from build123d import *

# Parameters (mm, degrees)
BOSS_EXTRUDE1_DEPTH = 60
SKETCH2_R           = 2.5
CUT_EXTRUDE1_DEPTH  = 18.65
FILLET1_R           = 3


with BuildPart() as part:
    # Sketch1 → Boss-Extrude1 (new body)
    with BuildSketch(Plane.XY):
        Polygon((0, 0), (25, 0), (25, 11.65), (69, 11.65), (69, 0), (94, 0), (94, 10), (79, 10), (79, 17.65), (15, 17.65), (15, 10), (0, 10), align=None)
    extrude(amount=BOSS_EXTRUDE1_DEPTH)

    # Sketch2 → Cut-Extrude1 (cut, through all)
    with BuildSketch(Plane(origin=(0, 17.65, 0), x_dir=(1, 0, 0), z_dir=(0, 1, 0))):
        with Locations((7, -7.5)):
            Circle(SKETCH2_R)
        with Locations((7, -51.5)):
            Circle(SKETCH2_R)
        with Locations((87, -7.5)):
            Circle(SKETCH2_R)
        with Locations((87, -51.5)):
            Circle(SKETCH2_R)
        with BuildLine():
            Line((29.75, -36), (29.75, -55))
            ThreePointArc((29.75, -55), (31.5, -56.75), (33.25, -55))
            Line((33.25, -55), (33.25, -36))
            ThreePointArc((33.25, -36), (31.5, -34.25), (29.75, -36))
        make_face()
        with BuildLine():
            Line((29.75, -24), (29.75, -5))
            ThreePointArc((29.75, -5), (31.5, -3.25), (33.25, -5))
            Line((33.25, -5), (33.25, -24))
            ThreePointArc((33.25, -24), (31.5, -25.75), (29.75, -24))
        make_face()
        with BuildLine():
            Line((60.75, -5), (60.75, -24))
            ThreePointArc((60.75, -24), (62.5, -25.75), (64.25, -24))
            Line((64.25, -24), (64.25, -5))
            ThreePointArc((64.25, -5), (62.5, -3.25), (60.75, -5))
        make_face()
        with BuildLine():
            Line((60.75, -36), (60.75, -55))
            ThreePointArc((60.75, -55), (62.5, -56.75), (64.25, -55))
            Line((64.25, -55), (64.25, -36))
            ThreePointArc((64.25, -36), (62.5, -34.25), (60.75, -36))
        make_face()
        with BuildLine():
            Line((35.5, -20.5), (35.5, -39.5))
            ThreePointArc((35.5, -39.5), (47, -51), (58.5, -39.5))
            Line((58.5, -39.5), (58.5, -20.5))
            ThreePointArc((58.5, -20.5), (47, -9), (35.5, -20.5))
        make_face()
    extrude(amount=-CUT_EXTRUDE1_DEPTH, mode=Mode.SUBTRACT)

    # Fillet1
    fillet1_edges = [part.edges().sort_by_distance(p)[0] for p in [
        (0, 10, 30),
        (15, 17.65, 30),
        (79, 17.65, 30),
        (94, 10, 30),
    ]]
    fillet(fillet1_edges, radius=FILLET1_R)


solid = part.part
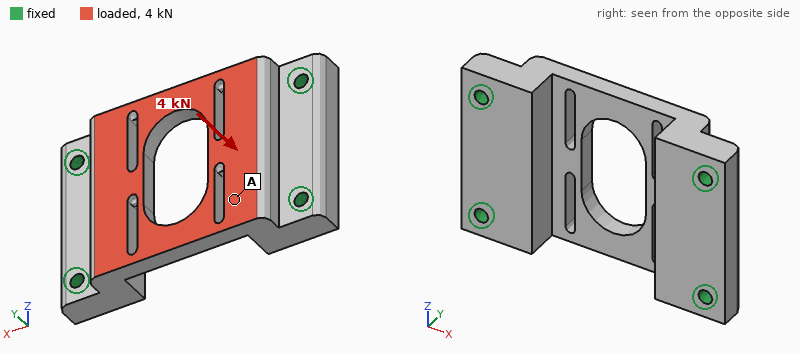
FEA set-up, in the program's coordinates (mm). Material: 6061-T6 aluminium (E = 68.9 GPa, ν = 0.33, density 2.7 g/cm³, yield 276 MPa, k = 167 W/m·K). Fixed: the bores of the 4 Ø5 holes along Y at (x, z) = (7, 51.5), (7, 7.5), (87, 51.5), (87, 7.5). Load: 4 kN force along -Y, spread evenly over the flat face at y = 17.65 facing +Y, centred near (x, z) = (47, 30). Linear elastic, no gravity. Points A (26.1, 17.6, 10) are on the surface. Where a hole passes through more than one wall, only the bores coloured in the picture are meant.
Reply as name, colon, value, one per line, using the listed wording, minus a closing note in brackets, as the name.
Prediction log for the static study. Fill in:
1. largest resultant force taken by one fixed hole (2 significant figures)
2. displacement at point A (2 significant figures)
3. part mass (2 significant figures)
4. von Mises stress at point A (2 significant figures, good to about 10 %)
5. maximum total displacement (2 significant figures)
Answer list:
largest resultant force taken by one fixed hole: 1.2 kN
displacement at point A: 22 µm
part mass: 130 g
von Mises stress at point A: 10 MPa
maximum total displacement: 56 µm
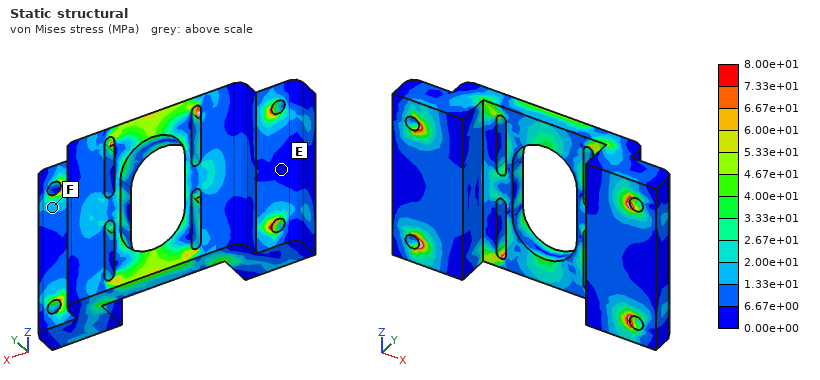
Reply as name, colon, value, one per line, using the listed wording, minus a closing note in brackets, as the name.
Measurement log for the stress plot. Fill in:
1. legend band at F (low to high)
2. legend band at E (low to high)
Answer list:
legend band at F: 1.33e+01 to 2.00e+01 MPa
legend band at E: 0.00e+00 to 6.67e+00 MPa
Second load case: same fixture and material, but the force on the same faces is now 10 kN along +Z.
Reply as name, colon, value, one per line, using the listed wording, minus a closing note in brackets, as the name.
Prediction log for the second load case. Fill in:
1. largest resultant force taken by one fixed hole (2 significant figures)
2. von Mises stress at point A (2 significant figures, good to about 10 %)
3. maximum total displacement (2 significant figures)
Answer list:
largest resultant force taken by one fixed hole: 3.5 kN
von Mises stress at point A: 26 MPa
maximum total displacement: 49 µm
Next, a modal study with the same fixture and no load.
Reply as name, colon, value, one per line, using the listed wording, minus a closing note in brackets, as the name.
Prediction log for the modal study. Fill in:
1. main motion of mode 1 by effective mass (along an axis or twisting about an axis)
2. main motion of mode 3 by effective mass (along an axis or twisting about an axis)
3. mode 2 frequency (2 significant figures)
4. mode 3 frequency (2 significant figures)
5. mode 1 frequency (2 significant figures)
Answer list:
main motion of mode 1 by effective mass: along Y
main motion of mode 3 by effective mass: twisting about X
mode 2 frequency: 8600 Hz
mode 3 frequency: 9400 Hz
mode 1 frequency: 7700 Hz
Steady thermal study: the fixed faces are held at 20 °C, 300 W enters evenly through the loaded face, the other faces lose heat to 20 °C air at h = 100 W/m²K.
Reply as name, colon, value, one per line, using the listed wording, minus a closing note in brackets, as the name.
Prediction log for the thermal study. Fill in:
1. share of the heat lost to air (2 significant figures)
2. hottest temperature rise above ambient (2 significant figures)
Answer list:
share of the heat lost to air: 12 %
hottest temperature rise above ambient: 82 K
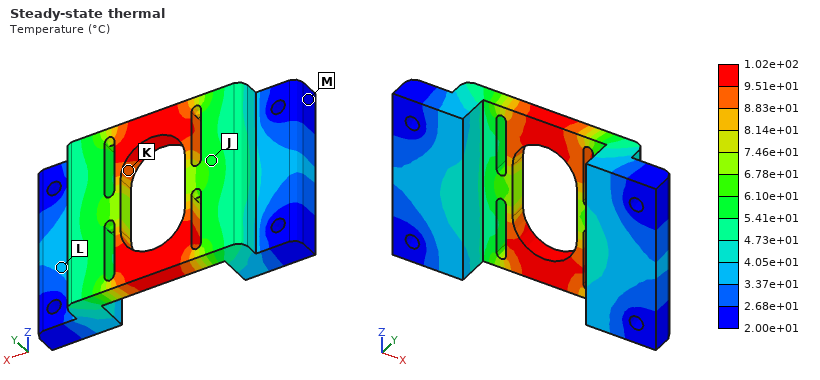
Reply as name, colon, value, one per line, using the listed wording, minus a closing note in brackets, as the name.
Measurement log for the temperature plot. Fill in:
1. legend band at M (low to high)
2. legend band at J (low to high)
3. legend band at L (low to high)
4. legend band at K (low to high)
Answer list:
legend band at M: 2.00e+01 to 2.68e+01 °C
legend band at J: 5.41e+01 to 6.10e+01 °C
legend band at L: 3.37e+01 to 4.05e+01 °C
legend band at K: 8.83e+01 to 9.51e+01 °C
